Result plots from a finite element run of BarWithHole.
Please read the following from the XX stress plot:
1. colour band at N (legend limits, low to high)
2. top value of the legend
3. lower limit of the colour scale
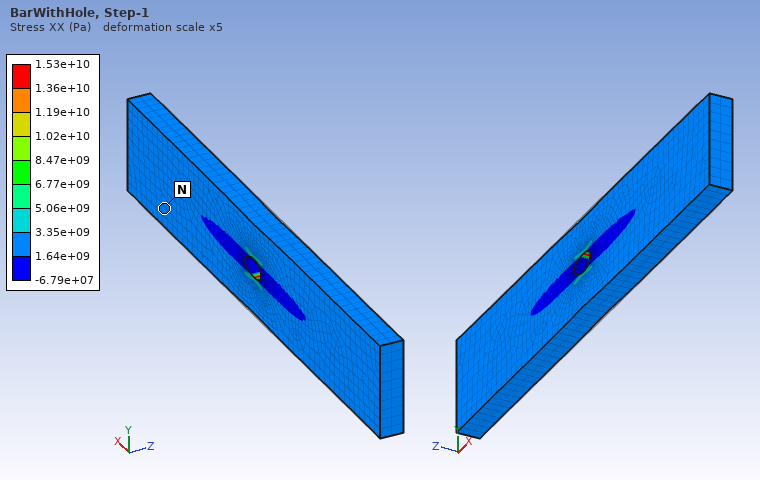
1.64e+09 to 3.35e+09 Pa
1.53e+10 Pa
-6.79e+07 Pa
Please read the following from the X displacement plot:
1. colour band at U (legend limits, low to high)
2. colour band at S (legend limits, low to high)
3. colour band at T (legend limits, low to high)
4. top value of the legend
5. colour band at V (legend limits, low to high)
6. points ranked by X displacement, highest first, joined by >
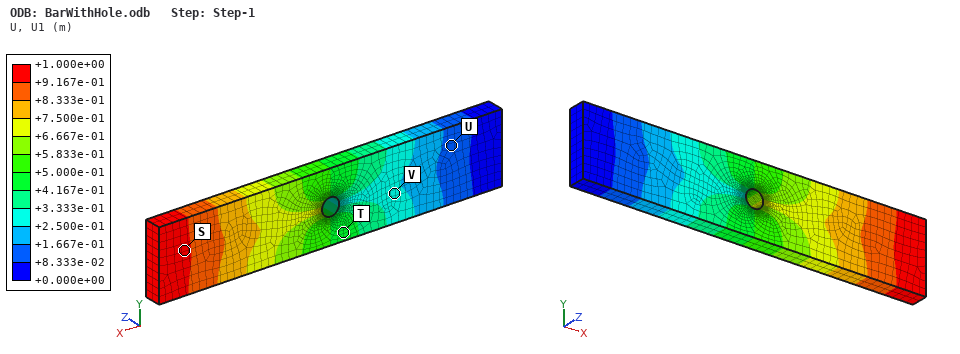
+8.333e-02 to +1.667e-01 m
+9.167e-01 to +1.000e+00 m
+4.167e-01 to +5.000e-01 m
+1.000e+00 m
+2.500e-01 to +3.333e-01 m
S > T > V > U
